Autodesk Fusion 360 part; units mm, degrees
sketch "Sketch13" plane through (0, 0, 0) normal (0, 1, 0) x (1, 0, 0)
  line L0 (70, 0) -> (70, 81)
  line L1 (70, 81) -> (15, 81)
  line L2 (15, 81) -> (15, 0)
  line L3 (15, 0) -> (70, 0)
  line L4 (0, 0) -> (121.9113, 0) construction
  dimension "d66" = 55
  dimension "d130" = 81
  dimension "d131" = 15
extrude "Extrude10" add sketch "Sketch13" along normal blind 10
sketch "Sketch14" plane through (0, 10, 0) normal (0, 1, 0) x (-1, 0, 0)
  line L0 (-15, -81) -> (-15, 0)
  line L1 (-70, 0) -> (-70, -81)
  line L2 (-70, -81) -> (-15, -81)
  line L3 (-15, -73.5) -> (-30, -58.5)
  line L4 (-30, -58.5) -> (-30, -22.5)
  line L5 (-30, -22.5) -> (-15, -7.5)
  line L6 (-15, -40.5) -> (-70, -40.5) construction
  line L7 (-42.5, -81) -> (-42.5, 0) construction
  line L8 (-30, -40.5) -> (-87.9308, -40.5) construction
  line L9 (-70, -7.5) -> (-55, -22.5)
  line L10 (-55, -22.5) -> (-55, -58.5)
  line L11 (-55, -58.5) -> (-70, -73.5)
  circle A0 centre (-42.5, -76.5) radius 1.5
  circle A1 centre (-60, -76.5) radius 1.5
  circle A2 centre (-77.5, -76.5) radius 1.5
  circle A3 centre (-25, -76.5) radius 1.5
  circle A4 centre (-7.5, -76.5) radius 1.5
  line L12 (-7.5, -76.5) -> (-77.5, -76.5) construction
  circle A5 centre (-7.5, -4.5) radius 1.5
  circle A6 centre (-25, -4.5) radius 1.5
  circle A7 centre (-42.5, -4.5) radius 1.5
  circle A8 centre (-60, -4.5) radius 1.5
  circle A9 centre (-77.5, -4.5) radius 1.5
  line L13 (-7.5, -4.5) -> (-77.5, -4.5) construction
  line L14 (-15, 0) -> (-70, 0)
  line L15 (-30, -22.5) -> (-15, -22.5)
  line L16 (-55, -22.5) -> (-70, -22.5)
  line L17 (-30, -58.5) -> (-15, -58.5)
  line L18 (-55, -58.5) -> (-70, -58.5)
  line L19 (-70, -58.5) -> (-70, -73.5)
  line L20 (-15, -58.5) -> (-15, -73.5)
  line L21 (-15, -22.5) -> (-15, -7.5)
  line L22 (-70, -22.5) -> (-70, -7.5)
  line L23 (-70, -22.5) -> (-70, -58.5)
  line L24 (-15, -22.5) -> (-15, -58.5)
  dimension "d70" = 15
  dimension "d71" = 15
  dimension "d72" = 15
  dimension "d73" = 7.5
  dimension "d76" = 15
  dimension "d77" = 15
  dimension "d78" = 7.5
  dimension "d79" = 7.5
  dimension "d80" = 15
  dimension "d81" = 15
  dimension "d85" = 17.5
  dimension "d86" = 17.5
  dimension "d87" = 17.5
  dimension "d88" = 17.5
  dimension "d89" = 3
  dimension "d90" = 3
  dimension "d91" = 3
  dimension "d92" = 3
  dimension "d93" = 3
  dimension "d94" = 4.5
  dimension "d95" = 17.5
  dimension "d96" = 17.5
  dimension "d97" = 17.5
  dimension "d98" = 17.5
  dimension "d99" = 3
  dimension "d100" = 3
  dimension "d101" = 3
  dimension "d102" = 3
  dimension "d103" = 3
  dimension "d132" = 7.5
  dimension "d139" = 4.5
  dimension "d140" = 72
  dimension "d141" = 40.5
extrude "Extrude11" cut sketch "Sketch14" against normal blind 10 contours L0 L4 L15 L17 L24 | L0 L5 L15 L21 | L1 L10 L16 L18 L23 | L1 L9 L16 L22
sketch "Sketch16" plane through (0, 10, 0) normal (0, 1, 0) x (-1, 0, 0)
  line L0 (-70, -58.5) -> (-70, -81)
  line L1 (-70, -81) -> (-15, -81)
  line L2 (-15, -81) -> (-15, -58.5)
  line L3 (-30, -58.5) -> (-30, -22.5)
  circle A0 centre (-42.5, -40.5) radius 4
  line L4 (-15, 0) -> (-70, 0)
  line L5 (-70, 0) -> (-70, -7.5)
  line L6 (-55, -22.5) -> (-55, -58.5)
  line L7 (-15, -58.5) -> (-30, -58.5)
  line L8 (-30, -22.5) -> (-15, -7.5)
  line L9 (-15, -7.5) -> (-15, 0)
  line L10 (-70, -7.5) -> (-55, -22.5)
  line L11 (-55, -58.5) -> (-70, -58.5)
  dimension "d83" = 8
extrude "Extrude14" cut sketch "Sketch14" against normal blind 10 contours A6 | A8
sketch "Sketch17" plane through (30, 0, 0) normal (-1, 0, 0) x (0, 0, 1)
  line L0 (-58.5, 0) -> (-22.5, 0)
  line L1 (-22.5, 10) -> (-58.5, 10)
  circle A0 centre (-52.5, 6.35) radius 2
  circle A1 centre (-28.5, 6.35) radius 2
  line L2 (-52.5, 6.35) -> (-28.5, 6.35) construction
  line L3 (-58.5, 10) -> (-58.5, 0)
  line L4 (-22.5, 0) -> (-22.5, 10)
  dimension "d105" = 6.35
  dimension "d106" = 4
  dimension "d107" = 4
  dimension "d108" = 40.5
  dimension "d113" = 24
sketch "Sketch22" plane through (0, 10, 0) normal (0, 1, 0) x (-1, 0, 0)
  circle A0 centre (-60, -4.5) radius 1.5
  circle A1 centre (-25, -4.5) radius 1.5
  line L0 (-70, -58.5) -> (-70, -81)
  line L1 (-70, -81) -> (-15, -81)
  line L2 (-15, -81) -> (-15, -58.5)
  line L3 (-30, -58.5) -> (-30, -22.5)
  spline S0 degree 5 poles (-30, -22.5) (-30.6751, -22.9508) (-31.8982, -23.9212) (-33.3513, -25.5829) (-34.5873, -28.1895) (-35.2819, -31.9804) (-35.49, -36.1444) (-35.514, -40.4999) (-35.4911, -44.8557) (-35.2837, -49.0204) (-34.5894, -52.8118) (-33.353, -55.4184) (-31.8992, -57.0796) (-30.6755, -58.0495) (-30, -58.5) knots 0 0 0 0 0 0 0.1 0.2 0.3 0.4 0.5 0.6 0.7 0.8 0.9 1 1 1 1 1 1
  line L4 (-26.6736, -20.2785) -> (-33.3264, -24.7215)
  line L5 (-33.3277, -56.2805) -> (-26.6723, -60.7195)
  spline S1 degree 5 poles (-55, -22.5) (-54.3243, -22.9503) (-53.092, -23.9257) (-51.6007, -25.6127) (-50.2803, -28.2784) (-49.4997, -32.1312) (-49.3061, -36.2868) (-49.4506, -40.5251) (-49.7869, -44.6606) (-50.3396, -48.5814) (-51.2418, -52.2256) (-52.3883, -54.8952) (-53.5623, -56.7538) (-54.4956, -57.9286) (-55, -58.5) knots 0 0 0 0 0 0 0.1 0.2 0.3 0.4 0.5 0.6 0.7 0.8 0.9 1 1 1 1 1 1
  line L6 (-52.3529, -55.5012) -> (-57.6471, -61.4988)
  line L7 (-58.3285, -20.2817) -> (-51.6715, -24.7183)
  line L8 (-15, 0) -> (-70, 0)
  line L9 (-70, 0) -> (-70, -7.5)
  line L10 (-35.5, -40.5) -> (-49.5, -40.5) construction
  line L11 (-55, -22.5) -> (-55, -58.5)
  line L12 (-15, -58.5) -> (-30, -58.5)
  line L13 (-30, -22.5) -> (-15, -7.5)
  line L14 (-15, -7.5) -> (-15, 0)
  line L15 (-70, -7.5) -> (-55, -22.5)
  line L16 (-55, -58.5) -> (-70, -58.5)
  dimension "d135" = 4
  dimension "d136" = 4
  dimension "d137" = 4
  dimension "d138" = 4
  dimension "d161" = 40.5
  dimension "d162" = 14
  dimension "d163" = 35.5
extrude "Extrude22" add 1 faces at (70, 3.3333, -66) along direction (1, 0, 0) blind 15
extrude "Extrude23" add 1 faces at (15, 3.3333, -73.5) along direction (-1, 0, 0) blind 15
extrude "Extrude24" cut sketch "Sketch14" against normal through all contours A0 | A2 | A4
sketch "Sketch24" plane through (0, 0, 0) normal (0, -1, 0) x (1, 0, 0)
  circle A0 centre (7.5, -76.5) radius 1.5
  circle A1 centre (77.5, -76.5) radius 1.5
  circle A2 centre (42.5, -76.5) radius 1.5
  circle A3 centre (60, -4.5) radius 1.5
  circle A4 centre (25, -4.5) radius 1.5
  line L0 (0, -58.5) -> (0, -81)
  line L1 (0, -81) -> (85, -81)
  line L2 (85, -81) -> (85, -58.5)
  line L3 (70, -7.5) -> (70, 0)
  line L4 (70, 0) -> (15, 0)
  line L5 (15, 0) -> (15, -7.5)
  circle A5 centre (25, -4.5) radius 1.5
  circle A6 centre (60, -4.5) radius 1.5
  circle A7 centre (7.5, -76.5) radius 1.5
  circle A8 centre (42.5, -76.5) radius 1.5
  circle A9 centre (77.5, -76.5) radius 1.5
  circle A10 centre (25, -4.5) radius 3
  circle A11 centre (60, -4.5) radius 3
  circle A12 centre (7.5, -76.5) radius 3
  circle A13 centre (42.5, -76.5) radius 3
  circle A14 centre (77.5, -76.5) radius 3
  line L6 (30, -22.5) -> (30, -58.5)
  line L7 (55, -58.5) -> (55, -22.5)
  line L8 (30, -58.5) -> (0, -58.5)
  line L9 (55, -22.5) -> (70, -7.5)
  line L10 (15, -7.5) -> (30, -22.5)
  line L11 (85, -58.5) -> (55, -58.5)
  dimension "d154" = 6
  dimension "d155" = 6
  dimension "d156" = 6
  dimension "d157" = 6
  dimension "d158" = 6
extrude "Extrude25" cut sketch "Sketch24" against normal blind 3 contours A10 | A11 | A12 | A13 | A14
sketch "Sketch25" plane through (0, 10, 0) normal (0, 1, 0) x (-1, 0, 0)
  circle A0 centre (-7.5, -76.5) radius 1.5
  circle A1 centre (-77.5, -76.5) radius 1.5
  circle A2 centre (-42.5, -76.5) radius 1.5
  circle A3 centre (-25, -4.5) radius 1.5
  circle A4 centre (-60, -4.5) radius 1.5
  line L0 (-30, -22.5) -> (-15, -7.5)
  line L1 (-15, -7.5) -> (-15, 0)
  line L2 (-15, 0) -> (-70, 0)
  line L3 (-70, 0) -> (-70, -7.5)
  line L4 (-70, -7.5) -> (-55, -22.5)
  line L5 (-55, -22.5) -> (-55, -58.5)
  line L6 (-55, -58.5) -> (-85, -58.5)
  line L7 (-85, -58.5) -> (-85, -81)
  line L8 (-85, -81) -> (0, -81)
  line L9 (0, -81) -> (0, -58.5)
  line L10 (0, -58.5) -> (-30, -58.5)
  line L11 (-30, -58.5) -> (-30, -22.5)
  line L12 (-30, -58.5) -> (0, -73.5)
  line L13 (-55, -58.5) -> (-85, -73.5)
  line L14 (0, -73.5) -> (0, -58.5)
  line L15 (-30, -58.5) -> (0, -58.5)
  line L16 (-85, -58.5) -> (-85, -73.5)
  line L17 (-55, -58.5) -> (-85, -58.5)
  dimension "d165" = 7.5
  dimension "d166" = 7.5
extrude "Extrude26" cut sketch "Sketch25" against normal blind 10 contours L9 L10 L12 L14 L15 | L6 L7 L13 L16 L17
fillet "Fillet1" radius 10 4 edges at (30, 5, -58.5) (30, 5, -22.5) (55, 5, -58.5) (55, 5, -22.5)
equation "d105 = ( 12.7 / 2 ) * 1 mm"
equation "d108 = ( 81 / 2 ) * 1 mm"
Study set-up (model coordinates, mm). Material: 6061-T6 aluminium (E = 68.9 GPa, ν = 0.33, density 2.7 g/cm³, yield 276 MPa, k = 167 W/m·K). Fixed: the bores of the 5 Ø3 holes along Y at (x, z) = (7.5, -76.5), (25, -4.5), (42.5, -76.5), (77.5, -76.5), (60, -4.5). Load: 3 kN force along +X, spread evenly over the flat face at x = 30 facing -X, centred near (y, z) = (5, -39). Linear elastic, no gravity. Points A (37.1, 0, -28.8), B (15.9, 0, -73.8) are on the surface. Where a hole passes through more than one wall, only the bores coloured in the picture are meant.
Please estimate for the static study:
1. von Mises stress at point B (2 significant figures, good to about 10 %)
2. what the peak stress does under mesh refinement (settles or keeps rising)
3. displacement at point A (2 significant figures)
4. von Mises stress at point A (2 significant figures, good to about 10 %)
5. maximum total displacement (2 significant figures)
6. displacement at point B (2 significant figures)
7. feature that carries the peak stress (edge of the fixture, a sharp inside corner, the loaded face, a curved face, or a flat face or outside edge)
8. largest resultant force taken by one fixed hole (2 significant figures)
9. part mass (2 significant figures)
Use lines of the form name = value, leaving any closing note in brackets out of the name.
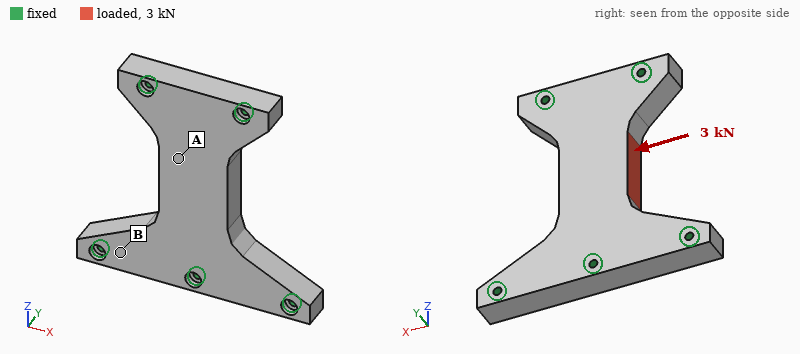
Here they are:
von Mises stress at point B = 4.6 MPa
what the peak stress does under mesh refinement = keeps rising
displacement at point A = 7.2 µm
von Mises stress at point A = 14 MPa
maximum total displacement = 10 µm
displacement at point B = 1.8 µm
feature that carries the peak stress = edge of the fixture
largest resultant force taken by one fixed hole = 1.2 kN
part mass = 90 g
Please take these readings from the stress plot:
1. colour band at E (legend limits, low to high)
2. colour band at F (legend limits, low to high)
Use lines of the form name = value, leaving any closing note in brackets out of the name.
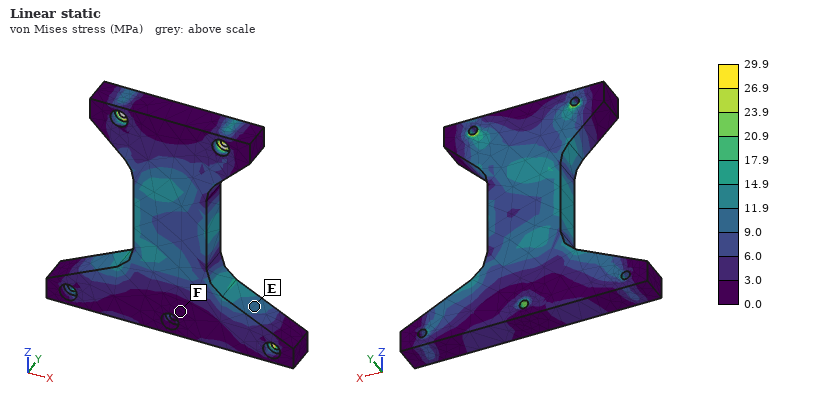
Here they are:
colour band at E = 9.0 to 11.9 MPa
colour band at F = 0.0 to 3.0 MPa
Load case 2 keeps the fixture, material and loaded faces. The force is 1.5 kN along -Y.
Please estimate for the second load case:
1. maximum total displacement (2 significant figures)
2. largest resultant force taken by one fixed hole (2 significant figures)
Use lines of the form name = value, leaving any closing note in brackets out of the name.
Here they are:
maximum total displacement = 48 µm
largest resultant force taken by one fixed hole = 710 N
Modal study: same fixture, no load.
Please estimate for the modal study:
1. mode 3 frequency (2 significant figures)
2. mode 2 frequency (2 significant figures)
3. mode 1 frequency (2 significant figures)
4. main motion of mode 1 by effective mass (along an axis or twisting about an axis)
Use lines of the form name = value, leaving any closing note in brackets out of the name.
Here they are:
mode 3 frequency = 16 kHz
mode 2 frequency = 16 kHz
mode 1 frequency = 7000 Hz
main motion of mode 1 by effective mass = along Y
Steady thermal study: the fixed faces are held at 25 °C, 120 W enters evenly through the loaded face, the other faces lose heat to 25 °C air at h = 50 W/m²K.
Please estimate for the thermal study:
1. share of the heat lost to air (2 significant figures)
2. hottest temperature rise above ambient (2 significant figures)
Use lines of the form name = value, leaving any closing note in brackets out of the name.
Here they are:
share of the heat lost to air = 5.7 %
hottest temperature rise above ambient = 59 K
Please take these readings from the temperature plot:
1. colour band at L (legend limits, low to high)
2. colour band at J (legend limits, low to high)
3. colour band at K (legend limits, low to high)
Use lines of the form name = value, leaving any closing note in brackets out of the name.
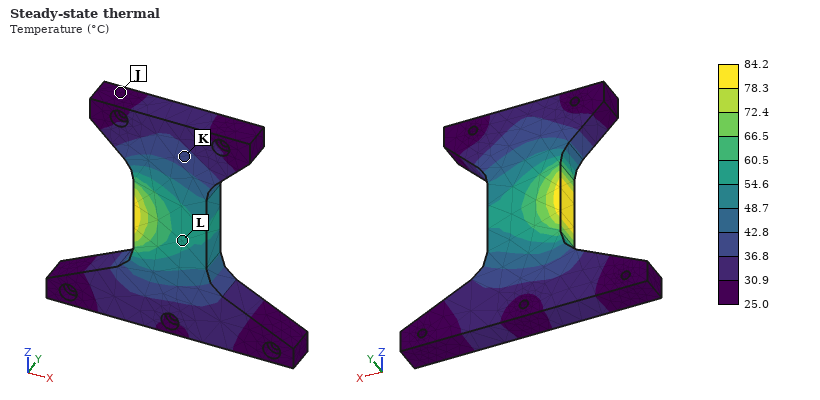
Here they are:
colour band at L = 54.6 to 60.5 °C
colour band at J = 25.0 to 30.9 °C
colour band at K = 36.8 to 42.8 °C
